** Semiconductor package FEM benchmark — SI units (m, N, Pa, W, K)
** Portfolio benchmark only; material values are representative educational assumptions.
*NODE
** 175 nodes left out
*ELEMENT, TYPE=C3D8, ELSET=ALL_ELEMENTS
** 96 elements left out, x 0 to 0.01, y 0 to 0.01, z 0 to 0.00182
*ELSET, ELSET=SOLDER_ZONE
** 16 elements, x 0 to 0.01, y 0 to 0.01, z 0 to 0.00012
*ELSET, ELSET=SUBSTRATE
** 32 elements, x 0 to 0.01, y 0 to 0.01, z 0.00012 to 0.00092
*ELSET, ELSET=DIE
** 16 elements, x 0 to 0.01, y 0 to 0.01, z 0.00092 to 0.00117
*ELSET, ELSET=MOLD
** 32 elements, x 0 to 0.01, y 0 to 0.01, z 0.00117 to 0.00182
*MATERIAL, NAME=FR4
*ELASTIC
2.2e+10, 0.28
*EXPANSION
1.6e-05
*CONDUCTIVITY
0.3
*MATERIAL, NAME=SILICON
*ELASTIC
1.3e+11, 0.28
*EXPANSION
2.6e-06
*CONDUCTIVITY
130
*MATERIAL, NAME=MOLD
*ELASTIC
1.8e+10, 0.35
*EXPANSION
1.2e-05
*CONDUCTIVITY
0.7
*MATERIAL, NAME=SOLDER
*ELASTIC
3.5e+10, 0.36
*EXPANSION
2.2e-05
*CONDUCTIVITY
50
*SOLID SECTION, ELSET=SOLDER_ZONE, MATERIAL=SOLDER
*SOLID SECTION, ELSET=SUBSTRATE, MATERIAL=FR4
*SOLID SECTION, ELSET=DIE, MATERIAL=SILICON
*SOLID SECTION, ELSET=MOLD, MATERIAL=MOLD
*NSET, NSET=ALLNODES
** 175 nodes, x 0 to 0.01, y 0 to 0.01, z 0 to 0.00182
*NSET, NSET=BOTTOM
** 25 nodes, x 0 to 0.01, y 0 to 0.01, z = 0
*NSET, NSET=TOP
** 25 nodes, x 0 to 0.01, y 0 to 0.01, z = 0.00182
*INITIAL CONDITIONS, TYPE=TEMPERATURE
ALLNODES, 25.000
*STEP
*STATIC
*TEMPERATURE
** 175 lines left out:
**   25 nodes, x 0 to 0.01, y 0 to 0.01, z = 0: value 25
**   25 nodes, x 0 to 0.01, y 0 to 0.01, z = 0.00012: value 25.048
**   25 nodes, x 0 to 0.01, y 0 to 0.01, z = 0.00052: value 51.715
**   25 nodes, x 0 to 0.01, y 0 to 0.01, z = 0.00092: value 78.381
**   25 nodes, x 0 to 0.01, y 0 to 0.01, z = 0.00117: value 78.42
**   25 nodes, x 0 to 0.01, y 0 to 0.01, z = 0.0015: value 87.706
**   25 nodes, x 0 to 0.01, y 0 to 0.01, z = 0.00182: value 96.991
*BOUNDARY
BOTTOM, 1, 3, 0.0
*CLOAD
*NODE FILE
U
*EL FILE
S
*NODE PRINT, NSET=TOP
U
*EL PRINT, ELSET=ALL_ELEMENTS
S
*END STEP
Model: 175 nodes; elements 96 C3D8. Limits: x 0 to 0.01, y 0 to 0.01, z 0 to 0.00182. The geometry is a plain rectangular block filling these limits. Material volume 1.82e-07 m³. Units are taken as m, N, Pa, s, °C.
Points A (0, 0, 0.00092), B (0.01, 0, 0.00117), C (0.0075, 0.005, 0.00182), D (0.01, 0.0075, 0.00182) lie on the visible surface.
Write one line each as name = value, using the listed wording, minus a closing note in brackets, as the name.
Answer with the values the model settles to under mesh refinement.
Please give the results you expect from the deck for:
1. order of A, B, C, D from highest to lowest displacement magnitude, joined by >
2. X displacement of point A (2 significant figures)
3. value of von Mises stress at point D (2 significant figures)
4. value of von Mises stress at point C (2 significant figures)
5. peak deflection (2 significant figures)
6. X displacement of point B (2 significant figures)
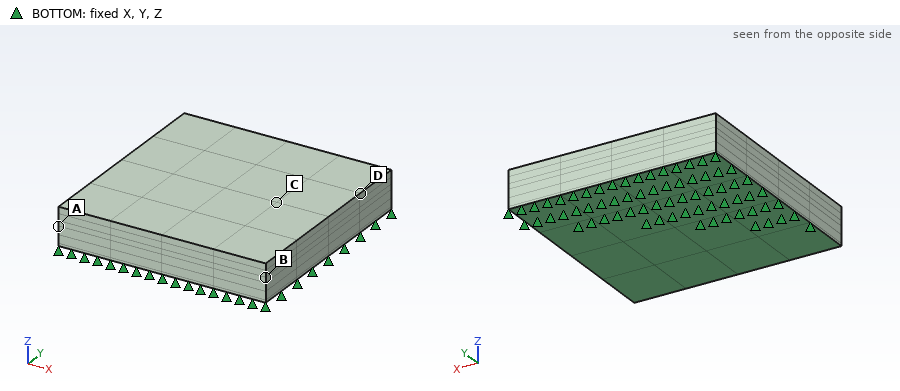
order of A, B, C, D from highest to lowest displacement magnitude, joined by > = D > C > B > A
X displacement of point A = -8.6e-07 m
value of von Mises stress at point D = 1.2e+07 Pa
value of von Mises stress at point C = 1.8e+07 Pa
peak deflection = 2.6e-06 m
X displacement of point B = 1.0e-06 m
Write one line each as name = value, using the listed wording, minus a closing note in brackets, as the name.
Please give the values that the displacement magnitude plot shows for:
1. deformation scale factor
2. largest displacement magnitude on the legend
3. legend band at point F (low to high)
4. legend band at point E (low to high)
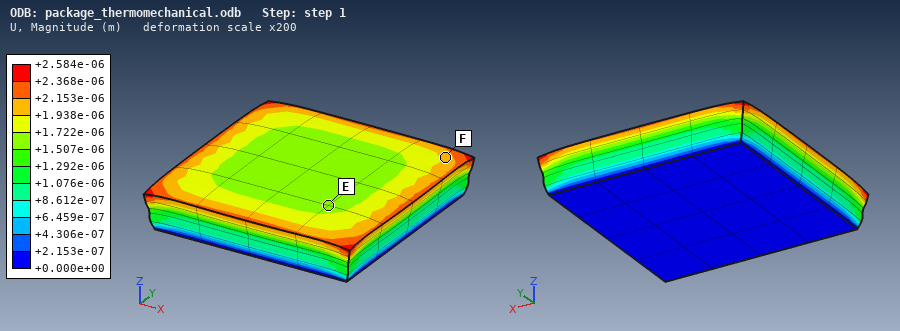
deformation scale factor = 200
largest displacement magnitude on the legend = +2.584e-06 m
legend band at point F = +1.938e-06 to +2.153e-06 m
legend band at point E = +1.507e-06 to +1.722e-06 m
